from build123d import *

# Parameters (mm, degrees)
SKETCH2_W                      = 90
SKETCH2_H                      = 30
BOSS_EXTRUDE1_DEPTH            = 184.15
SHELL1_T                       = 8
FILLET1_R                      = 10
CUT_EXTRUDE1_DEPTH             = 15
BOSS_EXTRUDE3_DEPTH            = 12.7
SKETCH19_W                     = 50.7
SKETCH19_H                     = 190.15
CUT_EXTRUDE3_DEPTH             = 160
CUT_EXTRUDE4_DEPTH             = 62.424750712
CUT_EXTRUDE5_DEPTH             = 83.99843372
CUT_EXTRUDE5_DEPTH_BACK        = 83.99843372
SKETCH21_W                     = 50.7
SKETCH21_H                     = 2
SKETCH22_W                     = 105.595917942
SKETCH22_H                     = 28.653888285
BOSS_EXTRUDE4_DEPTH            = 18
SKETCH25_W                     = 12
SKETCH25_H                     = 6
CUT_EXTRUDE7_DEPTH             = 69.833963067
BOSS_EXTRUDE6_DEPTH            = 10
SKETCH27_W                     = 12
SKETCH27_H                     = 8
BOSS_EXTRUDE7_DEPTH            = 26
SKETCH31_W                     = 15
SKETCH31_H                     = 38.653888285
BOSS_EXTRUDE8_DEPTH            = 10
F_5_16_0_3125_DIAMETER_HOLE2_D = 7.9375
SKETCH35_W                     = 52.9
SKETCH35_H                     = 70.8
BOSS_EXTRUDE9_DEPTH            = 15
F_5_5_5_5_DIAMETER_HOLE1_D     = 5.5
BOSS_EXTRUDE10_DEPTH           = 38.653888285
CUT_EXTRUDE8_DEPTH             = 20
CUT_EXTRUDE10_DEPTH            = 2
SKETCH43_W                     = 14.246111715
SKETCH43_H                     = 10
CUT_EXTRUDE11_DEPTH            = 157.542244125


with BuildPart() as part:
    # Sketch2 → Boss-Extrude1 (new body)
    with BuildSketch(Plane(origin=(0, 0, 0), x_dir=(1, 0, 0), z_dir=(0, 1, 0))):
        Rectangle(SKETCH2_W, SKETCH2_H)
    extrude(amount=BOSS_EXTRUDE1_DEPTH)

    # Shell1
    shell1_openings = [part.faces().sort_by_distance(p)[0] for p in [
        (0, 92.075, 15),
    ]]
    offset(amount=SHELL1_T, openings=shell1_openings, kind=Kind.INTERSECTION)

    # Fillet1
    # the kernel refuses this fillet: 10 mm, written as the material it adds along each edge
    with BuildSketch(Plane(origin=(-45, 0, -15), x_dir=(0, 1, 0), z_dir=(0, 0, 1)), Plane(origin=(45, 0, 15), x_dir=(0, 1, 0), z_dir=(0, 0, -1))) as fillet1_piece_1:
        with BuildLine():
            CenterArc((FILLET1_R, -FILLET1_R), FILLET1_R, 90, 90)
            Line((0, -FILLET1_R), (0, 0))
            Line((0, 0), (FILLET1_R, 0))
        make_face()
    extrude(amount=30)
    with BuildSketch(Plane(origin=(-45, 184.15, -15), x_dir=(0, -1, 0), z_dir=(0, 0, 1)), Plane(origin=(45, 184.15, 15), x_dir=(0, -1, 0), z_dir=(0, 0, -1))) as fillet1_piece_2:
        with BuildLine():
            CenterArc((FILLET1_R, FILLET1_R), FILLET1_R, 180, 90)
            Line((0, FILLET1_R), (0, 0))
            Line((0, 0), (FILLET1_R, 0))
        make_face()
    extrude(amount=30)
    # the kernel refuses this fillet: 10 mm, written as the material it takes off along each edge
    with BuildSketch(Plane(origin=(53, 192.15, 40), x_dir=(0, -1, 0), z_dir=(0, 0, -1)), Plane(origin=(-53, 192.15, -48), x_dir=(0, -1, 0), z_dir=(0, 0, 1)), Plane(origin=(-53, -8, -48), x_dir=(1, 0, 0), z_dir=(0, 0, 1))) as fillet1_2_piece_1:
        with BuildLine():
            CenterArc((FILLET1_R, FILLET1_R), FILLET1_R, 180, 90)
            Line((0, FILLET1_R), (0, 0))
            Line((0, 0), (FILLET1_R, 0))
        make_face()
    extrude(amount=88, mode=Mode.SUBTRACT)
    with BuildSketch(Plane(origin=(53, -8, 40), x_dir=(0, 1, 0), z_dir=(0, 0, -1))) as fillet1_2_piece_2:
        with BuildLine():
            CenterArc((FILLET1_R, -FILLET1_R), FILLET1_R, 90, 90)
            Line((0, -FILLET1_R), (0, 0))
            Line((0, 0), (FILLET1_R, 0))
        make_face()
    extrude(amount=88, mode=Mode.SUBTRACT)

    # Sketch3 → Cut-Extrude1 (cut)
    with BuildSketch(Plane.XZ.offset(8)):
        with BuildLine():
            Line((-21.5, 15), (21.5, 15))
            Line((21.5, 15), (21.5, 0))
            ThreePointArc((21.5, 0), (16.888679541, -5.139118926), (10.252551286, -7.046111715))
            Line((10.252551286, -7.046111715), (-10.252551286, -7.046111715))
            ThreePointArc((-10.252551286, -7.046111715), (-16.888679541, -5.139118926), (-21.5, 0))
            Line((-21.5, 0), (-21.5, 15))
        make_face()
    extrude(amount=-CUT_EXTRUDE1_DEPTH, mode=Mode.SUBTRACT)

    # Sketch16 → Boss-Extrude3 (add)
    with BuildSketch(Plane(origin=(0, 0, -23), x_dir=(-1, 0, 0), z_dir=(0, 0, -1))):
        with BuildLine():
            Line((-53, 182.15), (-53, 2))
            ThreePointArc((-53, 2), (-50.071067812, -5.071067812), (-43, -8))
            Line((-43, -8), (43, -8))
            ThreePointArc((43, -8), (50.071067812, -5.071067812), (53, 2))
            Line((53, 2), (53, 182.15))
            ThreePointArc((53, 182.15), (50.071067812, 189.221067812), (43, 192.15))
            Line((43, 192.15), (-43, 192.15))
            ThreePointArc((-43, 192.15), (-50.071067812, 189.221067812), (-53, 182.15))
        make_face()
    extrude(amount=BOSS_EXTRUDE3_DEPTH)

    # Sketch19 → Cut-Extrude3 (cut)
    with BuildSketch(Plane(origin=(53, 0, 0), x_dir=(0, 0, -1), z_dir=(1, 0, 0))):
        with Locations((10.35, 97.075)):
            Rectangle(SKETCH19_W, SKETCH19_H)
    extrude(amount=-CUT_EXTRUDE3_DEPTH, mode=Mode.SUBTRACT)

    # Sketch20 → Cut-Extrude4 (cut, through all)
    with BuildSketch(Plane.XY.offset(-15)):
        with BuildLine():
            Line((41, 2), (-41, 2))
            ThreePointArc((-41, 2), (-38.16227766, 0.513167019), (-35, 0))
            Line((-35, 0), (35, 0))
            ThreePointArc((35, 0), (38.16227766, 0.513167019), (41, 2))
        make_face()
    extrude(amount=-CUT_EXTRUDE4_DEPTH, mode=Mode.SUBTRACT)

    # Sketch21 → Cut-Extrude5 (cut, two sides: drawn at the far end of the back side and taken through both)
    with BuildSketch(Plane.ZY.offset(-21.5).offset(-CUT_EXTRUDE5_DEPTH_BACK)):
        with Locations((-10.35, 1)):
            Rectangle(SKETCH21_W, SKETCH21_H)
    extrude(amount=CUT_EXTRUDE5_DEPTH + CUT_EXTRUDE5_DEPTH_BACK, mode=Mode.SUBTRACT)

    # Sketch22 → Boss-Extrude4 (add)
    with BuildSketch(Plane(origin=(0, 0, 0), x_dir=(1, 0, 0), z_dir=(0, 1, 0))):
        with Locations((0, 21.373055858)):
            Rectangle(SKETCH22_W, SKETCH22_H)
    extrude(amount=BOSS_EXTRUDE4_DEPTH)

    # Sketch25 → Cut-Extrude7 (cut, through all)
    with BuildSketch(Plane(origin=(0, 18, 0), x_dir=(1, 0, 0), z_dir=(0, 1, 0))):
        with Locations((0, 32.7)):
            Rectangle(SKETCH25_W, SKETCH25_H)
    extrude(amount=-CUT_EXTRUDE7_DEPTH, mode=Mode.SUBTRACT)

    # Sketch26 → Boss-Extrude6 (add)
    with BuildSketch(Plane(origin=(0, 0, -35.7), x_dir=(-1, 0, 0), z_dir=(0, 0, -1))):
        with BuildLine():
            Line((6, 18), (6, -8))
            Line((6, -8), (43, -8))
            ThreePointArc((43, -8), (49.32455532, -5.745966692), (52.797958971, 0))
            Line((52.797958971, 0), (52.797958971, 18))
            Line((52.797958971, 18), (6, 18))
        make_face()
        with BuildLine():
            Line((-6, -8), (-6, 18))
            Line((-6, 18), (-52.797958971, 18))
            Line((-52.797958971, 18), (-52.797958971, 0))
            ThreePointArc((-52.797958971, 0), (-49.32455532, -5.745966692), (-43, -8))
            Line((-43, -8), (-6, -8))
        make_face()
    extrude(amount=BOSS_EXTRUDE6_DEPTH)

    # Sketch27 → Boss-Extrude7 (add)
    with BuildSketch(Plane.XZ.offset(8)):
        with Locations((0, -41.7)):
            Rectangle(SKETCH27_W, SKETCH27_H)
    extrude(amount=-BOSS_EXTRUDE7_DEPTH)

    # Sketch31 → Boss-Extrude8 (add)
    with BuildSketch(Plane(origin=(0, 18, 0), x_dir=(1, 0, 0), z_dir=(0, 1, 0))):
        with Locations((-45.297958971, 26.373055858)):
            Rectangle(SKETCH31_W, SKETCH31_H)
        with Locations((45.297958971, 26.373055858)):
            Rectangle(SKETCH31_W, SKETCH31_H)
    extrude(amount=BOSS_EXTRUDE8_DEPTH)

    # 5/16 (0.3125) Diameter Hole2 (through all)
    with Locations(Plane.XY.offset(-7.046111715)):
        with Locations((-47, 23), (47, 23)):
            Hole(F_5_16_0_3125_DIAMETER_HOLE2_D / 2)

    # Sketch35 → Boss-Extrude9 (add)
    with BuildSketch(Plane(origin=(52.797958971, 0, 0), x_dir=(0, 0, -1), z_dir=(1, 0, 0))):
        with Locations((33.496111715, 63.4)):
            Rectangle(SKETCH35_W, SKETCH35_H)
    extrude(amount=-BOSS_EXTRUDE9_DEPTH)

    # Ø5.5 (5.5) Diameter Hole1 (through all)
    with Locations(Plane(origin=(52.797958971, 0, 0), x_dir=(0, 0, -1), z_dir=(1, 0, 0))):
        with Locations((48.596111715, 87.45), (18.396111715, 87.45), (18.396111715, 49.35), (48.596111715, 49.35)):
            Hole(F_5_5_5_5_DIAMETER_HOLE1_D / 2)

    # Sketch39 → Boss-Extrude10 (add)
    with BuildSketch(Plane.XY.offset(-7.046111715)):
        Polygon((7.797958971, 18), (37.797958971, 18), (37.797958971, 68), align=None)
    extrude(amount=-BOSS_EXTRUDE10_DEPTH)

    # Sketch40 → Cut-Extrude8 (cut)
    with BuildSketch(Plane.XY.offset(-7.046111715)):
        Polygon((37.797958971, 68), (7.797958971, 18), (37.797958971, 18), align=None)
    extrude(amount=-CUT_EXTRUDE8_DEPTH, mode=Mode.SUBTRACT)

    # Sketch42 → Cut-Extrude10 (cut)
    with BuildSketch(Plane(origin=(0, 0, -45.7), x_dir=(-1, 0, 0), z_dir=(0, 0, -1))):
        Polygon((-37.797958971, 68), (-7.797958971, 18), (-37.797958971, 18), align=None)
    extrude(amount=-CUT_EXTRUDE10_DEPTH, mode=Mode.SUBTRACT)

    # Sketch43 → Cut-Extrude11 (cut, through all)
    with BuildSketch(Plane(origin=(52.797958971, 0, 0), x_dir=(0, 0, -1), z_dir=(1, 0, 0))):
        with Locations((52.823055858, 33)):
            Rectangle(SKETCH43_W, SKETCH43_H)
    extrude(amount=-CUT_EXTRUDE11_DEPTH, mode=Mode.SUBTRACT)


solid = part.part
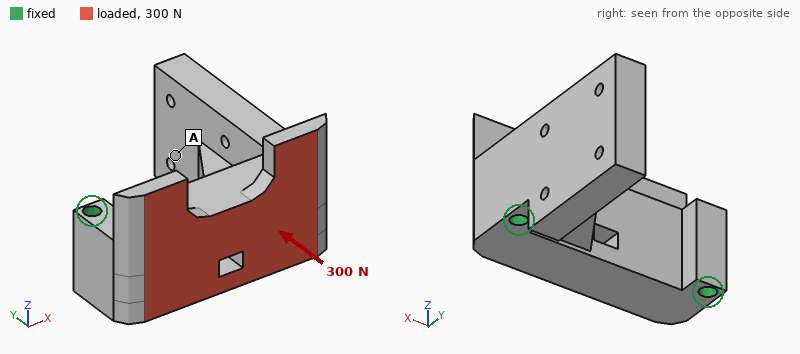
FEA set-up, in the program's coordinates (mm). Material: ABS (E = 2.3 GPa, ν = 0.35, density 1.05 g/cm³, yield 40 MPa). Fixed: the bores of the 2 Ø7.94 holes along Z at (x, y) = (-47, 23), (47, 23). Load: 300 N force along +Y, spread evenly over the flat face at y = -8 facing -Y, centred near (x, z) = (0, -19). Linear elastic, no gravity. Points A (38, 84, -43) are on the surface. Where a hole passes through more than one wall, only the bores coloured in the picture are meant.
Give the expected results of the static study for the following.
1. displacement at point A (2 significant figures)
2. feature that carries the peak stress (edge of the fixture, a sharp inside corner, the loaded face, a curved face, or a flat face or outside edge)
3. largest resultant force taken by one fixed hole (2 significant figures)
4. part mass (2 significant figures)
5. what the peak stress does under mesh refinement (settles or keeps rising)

13 µm
edge of the fixture
190 N
190 g
keeps rising
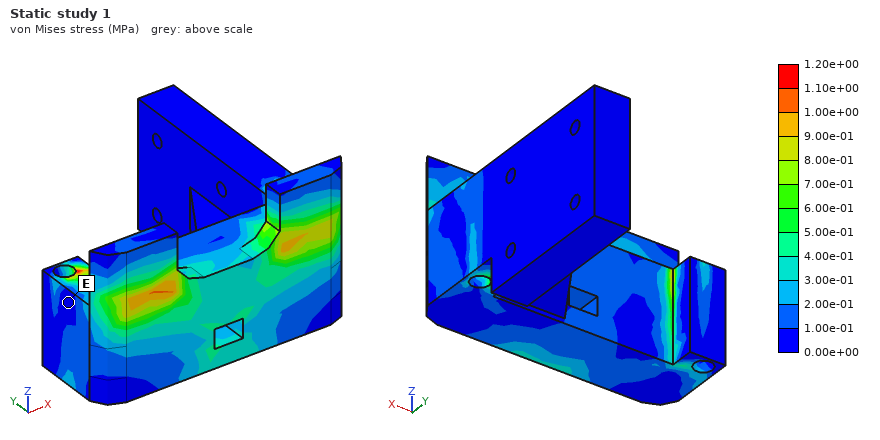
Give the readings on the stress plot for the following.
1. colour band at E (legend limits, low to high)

0.00e+00 to 1.00e-01 MPa
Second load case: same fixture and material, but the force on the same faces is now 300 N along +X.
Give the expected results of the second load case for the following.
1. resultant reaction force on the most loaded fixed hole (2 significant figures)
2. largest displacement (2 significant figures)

180 N
17 µm
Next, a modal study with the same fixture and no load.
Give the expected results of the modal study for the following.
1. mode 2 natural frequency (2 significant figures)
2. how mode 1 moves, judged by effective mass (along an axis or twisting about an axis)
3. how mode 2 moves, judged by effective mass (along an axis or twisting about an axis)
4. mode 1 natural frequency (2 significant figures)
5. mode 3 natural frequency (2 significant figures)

1300 Hz
along X
along Z
900 Hz
1700 Hz
